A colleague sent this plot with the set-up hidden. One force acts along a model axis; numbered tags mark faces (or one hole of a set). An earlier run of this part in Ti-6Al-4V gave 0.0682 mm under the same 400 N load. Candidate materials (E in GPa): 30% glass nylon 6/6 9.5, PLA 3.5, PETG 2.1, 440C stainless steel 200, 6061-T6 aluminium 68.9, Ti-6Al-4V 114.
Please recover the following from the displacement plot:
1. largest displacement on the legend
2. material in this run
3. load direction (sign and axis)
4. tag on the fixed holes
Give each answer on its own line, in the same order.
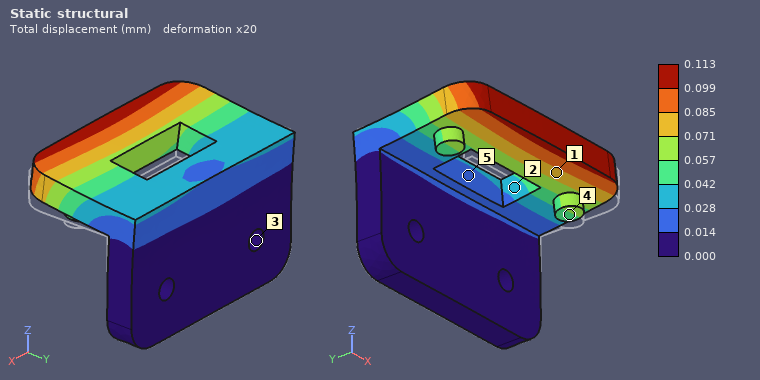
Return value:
0.113 mm
6061-T6 aluminium
+Z
3
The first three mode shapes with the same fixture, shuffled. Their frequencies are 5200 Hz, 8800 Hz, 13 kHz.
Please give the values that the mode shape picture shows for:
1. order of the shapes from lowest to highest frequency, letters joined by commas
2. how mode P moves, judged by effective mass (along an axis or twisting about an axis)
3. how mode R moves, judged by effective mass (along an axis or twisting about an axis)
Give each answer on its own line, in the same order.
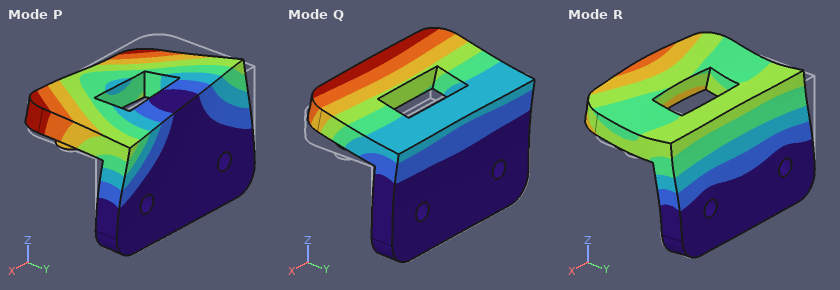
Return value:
Q, P, R
along X
along Y
